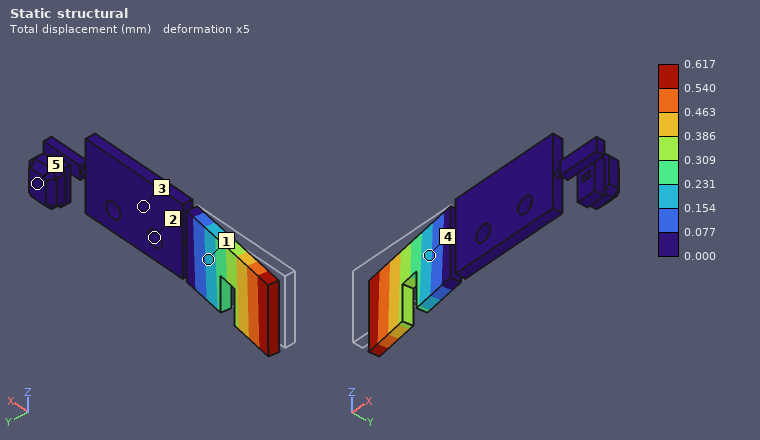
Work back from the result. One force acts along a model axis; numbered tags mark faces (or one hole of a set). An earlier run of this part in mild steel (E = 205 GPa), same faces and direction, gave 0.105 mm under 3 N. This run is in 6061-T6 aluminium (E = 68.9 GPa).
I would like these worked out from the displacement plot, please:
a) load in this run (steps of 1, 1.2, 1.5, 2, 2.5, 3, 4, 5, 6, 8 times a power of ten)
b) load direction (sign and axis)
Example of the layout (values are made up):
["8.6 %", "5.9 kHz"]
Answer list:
["6 N", "+Y"]
